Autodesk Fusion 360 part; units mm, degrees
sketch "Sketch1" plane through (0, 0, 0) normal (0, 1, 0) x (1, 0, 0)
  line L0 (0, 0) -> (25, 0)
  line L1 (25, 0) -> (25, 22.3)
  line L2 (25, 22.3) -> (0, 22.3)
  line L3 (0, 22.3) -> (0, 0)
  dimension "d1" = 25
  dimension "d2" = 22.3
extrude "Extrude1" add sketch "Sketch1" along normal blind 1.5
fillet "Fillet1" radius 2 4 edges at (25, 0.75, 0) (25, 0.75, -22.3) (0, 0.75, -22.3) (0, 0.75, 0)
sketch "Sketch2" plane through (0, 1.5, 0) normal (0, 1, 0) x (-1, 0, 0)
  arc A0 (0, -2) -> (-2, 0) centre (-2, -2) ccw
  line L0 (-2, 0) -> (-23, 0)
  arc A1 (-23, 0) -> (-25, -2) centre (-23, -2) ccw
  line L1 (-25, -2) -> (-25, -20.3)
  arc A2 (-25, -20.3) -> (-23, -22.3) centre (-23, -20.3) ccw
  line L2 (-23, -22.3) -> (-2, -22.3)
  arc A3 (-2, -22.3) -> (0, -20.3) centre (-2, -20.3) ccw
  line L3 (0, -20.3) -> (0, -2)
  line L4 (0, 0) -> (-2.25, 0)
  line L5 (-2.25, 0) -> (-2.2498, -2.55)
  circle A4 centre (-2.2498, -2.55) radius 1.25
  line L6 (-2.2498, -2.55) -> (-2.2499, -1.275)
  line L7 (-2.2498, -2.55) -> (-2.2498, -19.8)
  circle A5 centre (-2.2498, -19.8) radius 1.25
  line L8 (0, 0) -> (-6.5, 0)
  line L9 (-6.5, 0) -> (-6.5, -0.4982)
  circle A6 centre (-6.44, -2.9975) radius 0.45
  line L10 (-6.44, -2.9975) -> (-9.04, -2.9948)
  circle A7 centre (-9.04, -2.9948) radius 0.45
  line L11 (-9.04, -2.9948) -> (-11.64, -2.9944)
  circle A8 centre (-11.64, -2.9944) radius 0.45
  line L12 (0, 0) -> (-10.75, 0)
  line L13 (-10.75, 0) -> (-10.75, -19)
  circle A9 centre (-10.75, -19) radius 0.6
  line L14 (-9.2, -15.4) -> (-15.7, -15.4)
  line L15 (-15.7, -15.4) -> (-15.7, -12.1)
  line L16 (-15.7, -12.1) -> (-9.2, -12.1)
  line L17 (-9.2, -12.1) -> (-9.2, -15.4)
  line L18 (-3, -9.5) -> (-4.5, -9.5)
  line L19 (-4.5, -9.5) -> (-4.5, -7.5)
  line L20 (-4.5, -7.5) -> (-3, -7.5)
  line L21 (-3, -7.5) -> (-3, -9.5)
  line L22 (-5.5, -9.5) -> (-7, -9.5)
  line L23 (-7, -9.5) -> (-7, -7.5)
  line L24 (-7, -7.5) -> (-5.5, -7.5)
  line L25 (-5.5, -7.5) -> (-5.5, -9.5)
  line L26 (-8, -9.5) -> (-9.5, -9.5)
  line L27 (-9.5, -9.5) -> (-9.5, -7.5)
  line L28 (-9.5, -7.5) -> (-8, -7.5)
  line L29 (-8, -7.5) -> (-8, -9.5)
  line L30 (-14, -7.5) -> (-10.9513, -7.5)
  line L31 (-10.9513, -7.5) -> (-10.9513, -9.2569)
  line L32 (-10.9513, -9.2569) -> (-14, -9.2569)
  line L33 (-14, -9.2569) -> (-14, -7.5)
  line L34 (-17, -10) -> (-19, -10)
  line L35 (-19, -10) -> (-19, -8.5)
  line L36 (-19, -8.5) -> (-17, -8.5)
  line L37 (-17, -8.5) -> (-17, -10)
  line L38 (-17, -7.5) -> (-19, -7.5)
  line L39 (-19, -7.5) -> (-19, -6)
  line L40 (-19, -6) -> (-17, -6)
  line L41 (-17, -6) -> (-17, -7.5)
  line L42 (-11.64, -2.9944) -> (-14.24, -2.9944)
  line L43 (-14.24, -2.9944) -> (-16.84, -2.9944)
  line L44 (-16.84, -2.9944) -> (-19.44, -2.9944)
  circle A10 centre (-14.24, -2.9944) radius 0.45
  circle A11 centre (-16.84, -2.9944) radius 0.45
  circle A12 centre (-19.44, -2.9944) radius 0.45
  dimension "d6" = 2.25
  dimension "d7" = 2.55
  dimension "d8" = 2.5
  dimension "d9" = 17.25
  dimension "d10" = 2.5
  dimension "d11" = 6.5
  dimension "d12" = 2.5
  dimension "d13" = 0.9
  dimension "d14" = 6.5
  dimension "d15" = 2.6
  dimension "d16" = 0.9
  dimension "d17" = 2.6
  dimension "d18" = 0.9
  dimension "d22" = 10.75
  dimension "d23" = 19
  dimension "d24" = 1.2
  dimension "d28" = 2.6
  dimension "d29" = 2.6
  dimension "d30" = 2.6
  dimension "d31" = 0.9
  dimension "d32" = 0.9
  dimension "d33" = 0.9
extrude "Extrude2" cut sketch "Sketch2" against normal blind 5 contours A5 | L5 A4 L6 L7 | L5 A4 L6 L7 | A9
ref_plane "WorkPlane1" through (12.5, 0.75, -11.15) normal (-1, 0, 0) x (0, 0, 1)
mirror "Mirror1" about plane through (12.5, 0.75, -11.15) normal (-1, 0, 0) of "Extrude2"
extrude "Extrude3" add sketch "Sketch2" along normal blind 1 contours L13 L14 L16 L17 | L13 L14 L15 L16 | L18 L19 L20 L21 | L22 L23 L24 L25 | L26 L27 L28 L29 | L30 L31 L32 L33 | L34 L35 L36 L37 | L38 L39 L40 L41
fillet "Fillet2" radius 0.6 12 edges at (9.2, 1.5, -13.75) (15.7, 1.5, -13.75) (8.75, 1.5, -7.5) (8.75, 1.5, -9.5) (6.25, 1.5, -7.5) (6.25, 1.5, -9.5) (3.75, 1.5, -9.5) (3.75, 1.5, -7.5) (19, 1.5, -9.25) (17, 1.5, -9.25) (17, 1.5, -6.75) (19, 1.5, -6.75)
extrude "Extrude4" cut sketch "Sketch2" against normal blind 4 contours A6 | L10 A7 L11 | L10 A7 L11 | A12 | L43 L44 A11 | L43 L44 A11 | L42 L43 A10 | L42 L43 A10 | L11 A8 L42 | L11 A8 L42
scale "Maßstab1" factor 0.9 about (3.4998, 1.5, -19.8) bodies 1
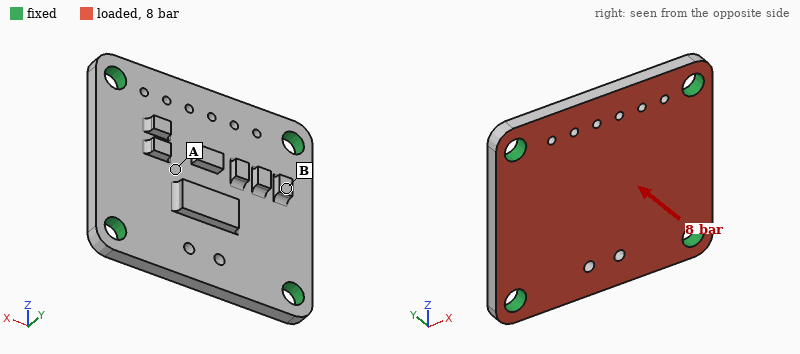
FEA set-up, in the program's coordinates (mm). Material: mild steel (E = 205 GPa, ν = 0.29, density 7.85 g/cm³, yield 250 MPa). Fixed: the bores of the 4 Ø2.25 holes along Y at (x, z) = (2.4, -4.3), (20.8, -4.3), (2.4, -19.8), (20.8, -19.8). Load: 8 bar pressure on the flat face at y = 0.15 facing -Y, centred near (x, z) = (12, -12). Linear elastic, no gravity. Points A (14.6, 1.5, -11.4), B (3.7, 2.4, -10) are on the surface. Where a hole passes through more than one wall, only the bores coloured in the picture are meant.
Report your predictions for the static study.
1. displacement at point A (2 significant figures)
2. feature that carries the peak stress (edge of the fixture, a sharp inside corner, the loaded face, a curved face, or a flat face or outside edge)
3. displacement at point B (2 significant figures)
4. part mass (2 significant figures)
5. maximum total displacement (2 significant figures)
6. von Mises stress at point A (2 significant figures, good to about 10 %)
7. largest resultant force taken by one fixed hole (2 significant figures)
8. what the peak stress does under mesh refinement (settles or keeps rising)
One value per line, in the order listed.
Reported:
7.1 µm
edge of the fixture
3.5 µm
4.8 g
7.7 µm
32 MPa
86 N
keeps rising
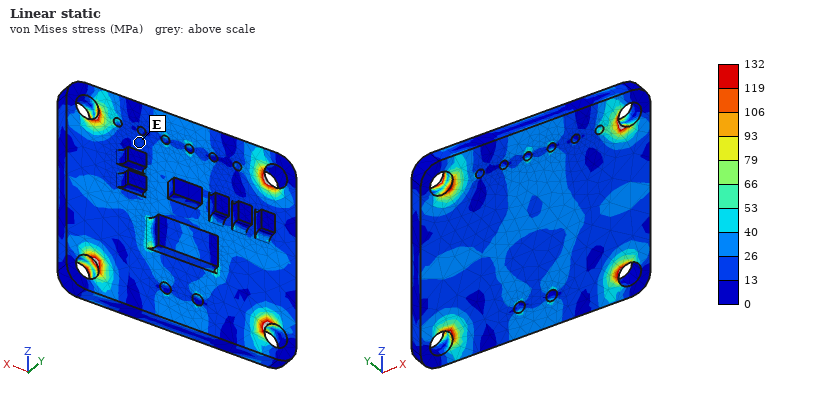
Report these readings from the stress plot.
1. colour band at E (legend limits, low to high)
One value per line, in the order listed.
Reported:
13 to 26 MPa
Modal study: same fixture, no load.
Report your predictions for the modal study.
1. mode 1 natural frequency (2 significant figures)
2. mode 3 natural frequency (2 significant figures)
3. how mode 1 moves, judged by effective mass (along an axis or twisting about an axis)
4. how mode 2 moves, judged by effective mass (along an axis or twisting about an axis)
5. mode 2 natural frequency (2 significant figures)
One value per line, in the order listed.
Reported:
18 kHz
33 kHz
along Y
twisting about X
27 kHz
